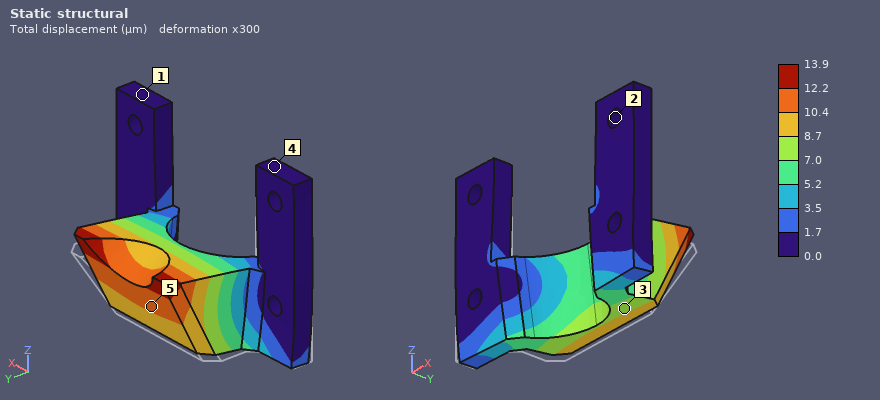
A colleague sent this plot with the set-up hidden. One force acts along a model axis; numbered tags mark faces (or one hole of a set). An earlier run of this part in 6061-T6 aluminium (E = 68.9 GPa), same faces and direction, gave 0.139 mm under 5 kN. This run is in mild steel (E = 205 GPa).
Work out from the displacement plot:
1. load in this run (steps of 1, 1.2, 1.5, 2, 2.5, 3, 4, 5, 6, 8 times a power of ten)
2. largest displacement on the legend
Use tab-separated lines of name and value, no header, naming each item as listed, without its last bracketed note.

load in this run	1.5 kN
largest displacement on the legend	13.9 µm
